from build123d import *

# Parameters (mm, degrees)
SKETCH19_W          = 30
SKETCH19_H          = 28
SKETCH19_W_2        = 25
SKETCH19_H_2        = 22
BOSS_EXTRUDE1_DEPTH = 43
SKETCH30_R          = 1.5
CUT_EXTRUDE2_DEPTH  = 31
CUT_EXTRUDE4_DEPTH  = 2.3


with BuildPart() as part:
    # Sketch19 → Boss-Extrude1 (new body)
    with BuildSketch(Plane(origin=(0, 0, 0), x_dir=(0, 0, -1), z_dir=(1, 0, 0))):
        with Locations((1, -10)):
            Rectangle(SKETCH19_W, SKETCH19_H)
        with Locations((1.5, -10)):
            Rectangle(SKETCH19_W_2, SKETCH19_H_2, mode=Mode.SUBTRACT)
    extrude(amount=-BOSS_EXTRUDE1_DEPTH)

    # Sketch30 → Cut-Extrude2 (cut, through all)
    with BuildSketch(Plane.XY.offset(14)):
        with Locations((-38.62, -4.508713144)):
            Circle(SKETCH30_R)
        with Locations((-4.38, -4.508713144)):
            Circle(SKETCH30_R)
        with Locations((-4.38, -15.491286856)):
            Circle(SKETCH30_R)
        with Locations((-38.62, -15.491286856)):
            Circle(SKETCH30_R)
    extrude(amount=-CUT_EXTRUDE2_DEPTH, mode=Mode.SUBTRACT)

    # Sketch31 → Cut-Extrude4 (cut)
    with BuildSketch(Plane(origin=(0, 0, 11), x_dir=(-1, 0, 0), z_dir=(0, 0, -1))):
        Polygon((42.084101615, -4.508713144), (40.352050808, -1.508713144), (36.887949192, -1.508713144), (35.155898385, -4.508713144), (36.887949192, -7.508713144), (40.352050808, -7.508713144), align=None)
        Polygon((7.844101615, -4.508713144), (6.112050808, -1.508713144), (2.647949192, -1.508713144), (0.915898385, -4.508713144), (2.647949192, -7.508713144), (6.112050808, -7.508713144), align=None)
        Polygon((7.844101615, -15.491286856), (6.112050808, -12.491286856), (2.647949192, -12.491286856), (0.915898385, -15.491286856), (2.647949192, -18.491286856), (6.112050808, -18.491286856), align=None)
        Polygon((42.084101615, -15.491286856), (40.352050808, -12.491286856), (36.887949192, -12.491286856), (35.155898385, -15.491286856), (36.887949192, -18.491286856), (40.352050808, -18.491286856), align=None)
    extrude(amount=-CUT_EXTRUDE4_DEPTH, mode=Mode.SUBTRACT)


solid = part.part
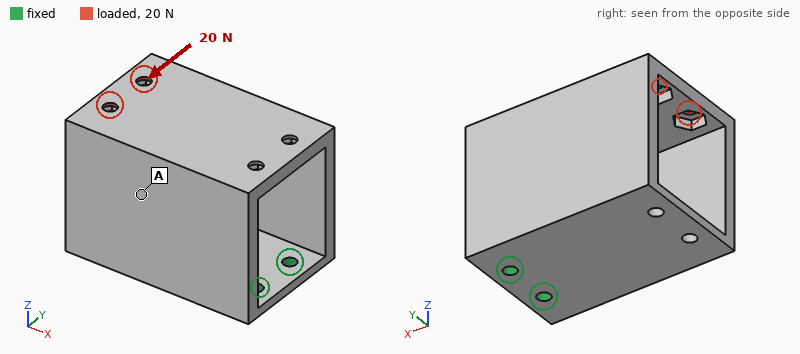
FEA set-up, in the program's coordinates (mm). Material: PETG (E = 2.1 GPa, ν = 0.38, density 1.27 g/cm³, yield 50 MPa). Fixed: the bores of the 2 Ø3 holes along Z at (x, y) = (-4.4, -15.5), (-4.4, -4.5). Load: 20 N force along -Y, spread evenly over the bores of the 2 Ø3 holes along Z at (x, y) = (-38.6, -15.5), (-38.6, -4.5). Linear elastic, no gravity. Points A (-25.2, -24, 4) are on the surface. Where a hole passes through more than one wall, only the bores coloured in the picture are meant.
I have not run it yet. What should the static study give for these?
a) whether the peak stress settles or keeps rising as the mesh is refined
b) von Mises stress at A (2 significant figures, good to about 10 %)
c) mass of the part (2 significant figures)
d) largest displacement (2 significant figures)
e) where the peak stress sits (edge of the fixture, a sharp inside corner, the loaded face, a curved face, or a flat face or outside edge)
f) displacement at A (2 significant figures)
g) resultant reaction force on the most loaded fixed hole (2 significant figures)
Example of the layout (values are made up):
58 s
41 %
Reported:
keeps rising
1.3 MPa
15 g
0.64 mm
edge of the fixture
0.47 mm
58 N
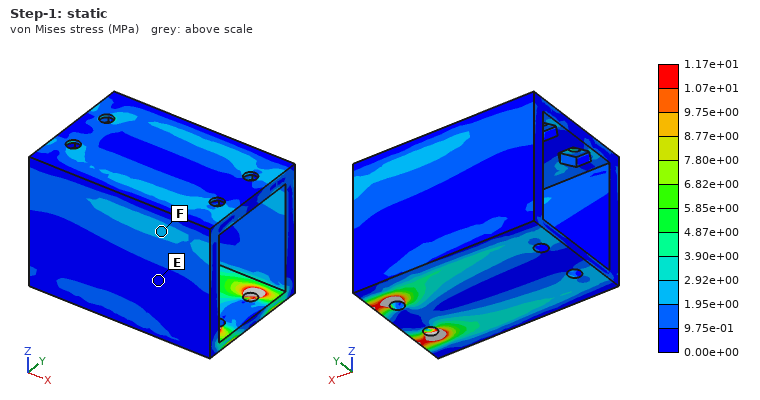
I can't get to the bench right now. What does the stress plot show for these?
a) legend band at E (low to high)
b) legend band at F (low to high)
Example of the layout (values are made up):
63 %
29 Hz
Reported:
0.00e+00 to 9.75e-01 MPa
1.95e+00 to 2.92e+00 MPa
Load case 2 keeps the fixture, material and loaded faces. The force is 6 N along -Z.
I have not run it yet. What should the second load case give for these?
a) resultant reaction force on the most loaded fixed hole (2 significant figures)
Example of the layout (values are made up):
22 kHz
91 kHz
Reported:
3.2 N
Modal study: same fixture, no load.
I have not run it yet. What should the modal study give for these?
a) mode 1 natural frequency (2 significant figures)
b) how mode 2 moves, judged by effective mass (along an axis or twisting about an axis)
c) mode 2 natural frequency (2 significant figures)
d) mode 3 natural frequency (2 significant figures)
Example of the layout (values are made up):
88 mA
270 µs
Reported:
180 Hz
along Y
320 Hz
840 Hz
